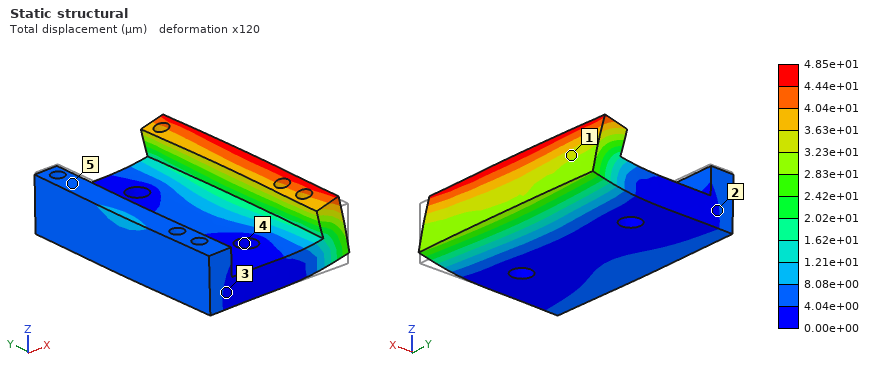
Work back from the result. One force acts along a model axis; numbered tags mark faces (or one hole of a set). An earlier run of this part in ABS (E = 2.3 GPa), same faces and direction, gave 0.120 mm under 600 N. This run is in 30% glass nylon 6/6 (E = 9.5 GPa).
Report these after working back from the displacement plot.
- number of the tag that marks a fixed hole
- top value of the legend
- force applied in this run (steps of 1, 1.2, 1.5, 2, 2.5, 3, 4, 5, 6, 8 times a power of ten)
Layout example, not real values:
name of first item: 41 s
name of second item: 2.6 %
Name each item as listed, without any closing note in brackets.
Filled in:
number of the tag that marks a fixed hole: 4
top value of the legend: 4.85e+01 µm
force applied in this run: 1 kN
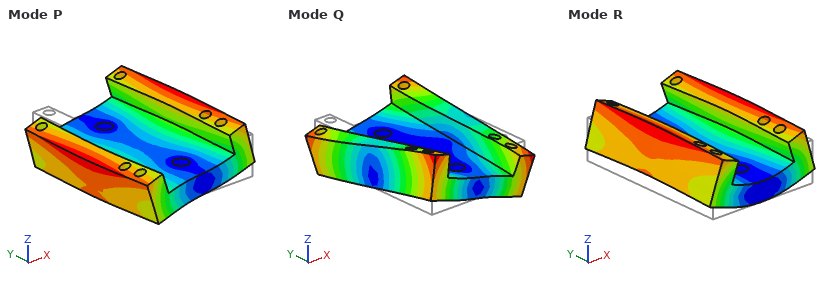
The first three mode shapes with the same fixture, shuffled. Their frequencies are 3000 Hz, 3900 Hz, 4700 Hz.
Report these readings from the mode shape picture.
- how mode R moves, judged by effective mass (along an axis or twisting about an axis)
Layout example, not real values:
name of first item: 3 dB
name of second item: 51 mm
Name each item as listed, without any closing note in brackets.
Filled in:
how mode R moves, judged by effective mass: along Z
